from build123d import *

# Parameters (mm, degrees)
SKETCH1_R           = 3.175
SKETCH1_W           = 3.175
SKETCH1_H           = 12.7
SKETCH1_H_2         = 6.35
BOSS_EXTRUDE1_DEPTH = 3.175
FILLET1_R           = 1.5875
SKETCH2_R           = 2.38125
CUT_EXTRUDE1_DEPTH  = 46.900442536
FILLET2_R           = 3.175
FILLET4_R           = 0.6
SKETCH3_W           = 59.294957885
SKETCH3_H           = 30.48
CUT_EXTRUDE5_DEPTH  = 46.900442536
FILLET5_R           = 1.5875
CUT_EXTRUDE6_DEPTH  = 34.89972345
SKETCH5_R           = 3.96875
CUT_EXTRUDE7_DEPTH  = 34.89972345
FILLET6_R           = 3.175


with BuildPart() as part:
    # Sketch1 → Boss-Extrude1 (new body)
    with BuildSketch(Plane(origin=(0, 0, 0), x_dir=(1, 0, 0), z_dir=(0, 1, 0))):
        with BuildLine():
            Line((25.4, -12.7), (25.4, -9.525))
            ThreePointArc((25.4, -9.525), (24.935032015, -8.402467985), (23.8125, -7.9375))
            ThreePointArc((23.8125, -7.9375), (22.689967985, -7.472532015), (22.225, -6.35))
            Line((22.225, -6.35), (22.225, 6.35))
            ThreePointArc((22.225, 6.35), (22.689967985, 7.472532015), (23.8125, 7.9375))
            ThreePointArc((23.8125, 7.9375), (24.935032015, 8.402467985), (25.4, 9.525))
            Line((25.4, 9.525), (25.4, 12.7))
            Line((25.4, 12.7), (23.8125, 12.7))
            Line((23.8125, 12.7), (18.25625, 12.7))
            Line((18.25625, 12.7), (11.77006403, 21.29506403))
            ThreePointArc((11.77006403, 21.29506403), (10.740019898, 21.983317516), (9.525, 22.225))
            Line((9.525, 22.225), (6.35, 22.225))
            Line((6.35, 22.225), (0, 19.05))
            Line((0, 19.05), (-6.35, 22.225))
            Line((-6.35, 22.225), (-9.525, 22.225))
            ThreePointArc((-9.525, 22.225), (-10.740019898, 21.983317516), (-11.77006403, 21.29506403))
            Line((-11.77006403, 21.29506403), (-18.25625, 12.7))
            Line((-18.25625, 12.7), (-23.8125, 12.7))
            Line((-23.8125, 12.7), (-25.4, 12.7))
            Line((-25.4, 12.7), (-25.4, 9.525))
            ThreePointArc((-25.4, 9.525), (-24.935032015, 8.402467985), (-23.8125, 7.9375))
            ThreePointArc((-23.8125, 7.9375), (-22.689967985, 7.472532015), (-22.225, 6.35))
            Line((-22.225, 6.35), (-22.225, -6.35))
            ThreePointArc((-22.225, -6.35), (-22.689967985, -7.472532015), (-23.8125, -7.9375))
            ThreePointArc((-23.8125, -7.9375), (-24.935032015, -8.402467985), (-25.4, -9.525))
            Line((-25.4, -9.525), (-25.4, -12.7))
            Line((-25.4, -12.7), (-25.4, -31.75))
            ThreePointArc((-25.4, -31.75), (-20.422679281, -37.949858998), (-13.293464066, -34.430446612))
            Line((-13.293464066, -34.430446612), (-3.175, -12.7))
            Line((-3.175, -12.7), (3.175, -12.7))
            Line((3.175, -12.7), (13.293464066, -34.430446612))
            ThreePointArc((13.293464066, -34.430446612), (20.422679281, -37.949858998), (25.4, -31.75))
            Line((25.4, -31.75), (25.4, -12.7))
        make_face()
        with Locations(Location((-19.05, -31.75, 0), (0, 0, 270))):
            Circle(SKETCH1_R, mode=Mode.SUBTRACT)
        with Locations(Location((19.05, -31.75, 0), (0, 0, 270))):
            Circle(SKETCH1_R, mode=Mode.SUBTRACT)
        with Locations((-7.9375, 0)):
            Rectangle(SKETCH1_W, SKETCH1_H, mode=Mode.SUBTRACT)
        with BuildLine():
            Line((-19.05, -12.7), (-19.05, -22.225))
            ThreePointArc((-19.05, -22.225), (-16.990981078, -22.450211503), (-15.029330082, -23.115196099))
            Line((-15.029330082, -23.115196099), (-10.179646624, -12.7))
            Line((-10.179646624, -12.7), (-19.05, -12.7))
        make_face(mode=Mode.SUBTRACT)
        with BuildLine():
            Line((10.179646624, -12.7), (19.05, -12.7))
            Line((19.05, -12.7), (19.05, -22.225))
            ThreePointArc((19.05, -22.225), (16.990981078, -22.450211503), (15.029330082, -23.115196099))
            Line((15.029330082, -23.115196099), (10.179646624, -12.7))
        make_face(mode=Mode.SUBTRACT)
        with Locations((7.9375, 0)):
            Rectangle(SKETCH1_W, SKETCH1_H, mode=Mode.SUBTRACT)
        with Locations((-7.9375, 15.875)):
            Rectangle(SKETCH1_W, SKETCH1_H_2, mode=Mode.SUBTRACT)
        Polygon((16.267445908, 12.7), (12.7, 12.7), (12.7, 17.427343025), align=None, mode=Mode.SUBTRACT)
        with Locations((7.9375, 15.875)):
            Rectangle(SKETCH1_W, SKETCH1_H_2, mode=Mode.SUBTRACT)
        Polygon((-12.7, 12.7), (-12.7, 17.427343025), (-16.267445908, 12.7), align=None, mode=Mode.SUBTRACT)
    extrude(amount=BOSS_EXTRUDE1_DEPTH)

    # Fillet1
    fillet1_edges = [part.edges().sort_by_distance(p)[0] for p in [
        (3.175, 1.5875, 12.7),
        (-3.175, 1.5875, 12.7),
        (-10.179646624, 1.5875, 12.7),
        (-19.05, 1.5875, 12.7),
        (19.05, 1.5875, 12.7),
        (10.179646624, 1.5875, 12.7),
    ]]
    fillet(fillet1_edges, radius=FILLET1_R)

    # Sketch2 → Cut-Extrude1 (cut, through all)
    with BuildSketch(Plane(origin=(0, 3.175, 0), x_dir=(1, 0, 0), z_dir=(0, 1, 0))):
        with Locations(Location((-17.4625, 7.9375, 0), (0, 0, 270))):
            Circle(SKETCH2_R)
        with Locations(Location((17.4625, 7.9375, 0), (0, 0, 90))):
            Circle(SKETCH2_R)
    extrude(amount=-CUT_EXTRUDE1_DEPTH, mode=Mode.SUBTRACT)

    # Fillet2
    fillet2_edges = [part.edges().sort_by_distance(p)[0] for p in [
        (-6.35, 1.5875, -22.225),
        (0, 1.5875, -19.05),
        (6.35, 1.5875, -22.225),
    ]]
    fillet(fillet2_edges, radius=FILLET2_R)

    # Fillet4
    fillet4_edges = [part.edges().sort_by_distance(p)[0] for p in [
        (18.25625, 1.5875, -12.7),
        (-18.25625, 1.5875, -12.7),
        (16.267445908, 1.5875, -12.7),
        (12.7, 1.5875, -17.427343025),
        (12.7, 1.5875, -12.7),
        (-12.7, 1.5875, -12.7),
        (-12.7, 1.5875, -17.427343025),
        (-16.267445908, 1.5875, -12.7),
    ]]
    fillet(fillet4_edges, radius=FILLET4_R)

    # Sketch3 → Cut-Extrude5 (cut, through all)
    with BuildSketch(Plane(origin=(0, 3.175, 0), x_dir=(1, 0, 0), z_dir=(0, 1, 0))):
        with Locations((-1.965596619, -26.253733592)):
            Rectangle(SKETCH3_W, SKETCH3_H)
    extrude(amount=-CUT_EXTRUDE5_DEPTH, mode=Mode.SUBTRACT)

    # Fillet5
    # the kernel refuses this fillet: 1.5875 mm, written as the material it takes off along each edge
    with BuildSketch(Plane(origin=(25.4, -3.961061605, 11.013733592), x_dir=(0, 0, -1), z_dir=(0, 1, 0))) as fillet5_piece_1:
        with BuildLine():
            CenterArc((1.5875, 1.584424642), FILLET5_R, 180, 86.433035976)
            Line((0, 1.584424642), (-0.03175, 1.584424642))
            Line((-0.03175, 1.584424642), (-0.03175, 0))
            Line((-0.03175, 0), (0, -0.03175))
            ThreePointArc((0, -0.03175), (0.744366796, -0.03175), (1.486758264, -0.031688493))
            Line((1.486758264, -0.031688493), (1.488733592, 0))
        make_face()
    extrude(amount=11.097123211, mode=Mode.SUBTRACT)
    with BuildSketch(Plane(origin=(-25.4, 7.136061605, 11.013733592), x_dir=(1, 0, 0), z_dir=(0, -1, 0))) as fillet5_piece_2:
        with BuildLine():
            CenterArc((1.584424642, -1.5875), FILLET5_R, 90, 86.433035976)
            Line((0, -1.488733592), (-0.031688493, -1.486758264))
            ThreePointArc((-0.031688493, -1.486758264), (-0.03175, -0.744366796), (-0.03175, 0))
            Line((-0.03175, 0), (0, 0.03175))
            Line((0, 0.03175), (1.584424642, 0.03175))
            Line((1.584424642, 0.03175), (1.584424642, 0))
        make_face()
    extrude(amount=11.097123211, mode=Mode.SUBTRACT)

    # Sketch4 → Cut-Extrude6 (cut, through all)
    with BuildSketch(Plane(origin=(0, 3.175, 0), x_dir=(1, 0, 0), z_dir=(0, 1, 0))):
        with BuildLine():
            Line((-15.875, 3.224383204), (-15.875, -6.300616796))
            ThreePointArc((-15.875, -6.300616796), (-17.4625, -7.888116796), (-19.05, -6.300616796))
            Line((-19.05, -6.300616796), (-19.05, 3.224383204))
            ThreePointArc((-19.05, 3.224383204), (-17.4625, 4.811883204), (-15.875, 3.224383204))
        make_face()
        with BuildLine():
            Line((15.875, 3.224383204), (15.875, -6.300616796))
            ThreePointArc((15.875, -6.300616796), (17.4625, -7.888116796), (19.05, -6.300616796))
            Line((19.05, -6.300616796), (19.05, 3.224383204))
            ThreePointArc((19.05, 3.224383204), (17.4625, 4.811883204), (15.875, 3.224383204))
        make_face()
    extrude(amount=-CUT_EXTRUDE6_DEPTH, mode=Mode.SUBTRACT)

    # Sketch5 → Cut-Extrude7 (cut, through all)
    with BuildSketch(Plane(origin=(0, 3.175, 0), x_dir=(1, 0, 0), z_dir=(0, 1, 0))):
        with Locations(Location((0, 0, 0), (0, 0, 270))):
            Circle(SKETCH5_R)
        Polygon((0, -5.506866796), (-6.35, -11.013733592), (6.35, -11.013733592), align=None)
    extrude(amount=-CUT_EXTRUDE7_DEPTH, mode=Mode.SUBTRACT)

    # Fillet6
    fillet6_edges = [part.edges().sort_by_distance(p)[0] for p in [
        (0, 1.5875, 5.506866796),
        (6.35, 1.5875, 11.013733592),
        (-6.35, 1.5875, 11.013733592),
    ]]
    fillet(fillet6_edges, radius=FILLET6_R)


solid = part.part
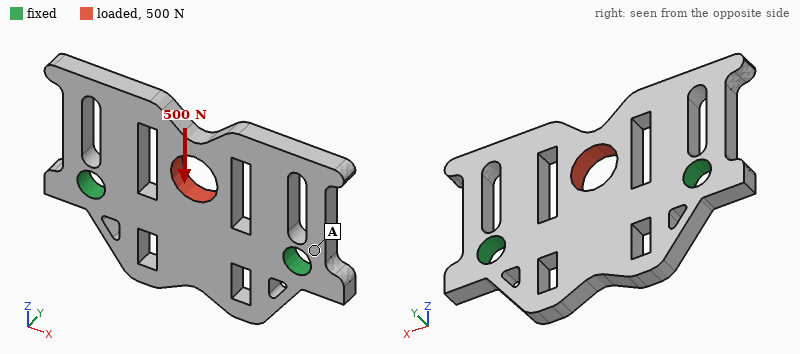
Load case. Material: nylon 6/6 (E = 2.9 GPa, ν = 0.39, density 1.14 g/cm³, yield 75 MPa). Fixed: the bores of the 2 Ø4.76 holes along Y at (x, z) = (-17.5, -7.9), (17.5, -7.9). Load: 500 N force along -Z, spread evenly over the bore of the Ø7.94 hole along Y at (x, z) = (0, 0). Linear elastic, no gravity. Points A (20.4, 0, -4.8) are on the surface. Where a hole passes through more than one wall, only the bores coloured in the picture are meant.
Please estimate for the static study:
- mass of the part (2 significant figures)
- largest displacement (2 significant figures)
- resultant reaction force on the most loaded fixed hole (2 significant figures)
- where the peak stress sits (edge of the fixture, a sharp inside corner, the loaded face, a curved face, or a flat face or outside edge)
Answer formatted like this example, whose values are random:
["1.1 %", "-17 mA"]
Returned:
["3.7 g", "0.27 mm", "250 N", "a curved face"]
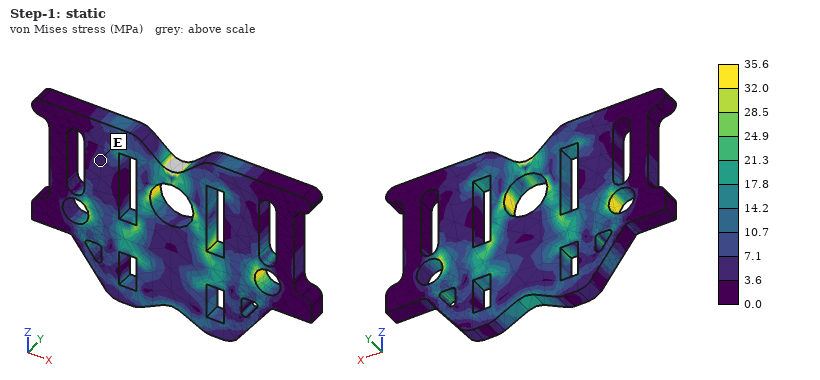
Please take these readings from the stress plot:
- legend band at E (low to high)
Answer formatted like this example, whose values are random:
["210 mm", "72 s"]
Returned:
["3.6 to 7.1 MPa"]
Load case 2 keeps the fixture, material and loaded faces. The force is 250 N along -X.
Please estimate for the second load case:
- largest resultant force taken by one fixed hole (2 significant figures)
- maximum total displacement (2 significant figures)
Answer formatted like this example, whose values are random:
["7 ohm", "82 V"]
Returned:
["140 N", "0.11 mm"]
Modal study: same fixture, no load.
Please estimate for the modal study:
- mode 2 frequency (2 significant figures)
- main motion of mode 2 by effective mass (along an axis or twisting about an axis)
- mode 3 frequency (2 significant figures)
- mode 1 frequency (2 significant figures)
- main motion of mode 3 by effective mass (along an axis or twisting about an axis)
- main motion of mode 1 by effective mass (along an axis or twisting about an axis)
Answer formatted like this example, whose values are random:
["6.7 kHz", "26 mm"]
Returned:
["2500 Hz", "twisting about Z", "3200 Hz", "1800 Hz", "along Y", "along Y"]
